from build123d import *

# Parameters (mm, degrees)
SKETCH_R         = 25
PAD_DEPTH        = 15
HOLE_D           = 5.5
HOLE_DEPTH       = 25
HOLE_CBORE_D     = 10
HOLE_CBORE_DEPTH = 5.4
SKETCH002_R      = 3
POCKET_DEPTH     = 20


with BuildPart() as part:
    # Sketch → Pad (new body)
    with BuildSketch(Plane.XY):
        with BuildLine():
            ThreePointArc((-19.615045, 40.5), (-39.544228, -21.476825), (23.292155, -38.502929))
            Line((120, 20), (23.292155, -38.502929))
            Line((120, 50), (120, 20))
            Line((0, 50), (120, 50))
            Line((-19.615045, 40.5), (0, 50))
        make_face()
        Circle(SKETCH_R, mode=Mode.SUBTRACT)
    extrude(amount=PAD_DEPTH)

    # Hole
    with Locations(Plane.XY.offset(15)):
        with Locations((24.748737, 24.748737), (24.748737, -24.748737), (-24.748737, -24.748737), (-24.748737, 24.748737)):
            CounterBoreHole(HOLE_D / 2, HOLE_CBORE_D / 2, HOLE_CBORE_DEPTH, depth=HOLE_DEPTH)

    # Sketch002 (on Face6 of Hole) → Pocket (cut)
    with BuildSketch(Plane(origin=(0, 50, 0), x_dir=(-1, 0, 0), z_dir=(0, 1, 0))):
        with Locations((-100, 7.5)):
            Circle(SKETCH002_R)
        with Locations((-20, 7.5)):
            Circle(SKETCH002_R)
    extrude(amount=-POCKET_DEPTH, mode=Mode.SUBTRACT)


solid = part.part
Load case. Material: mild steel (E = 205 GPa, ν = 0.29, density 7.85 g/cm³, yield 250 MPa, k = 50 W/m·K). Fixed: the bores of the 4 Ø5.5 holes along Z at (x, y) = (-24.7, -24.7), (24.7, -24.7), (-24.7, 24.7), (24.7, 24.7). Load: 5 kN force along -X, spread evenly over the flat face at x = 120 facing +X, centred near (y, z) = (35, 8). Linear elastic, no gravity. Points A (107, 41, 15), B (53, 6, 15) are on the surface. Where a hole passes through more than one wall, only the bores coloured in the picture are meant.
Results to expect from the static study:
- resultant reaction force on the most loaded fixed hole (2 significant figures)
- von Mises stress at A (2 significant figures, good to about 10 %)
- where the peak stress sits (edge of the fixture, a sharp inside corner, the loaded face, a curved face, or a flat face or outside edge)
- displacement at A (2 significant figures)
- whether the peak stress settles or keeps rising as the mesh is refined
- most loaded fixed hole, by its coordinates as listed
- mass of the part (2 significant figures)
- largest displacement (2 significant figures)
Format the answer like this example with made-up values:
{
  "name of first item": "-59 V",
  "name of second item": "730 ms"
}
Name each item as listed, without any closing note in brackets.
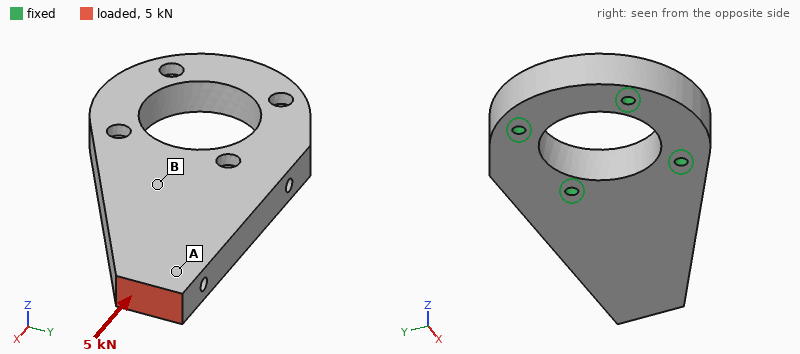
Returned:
{
  "resultant reaction force on the most loaded fixed hole": "4.2 kN",
  "von Mises stress at A": "16 MPa",
  "where the peak stress sits": "edge of the fixture",
  "displacement at A": "9.9 µm",
  "whether the peak stress settles or keeps rising as the mesh is refined": "keeps rising",
  "most loaded fixed hole, by its coordinates as listed": "(24.7, 24.7)",
  "mass of the part": "1.0 kg",
  "largest displacement": "13 µm"
}
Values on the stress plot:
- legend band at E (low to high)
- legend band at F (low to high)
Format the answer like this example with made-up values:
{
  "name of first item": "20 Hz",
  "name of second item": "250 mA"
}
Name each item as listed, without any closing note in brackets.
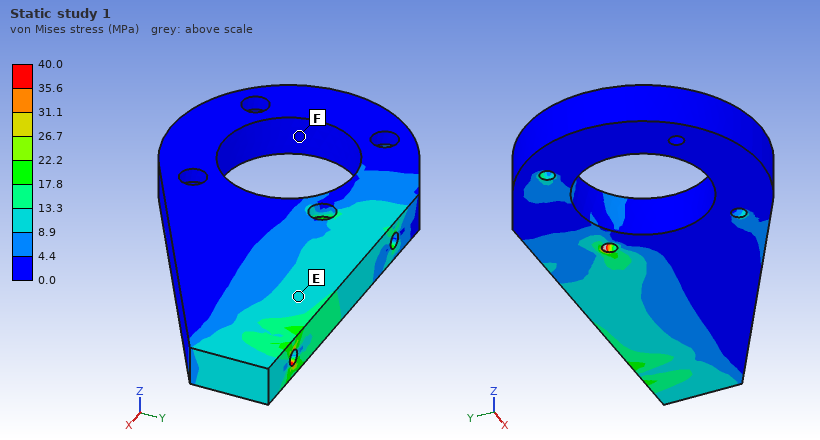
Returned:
{
  "legend band at E": "8.9 to 13.3 MPa",
  "legend band at F": "0.0 to 4.4 MPa"
}
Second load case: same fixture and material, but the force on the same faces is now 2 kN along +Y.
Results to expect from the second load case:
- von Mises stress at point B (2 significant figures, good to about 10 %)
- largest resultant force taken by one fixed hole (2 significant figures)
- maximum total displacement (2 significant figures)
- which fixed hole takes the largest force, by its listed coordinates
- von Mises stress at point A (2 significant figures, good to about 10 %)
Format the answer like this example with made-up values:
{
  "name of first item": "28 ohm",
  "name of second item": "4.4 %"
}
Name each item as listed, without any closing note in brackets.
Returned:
{
  "von Mises stress at point B": "4.0 MPa",
  "largest resultant force taken by one fixed hole": "3.5 kN",
  "maximum total displacement": "17 µm",
  "which fixed hole takes the largest force, by its listed coordinates": "(24.7, -24.7)",
  "von Mises stress at point A": "7.2 MPa"
}
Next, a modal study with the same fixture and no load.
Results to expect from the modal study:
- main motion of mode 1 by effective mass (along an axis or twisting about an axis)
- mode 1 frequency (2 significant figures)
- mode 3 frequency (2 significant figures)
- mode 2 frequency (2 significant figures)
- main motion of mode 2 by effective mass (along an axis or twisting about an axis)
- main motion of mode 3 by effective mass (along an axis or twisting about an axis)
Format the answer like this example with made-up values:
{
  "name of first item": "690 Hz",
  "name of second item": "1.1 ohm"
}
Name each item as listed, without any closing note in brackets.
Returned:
{
  "main motion of mode 1 by effective mass": "along Z",
  "mode 1 frequency": "1300 Hz",
  "mode 3 frequency": "5300 Hz",
  "mode 2 frequency": "5100 Hz",
  "main motion of mode 2 by effective mass": "along Y",
  "main motion of mode 3 by effective mass": "along Y"
}
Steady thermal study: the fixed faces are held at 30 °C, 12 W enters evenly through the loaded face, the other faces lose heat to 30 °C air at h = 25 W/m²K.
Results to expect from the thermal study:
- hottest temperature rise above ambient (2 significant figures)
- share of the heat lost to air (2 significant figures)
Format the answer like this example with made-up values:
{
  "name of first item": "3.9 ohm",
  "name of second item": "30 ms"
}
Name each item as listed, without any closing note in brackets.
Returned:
{
  "hottest temperature rise above ambient": "29 K",
  "share of the heat lost to air": "33 %"
}
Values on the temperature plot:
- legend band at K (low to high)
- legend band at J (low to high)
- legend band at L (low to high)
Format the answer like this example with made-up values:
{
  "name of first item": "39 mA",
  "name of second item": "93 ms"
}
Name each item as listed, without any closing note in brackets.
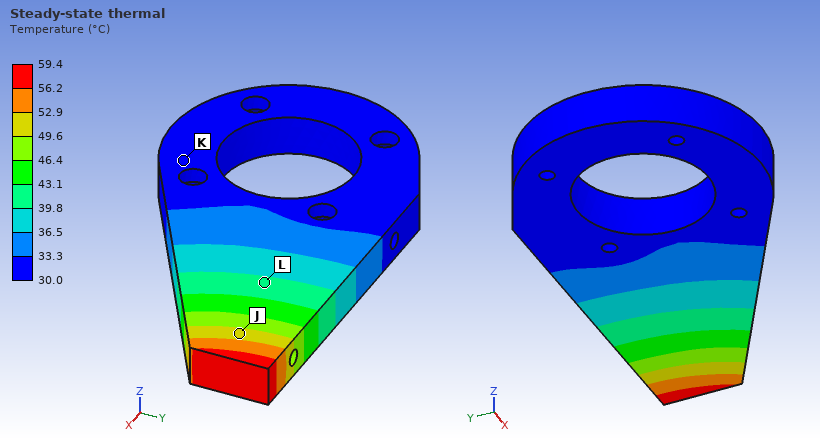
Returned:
{
  "legend band at K": "30.0 to 33.3 °C",
  "legend band at J": "49.6 to 52.9 °C",
  "legend band at L": "39.8 to 43.1 °C"
}
